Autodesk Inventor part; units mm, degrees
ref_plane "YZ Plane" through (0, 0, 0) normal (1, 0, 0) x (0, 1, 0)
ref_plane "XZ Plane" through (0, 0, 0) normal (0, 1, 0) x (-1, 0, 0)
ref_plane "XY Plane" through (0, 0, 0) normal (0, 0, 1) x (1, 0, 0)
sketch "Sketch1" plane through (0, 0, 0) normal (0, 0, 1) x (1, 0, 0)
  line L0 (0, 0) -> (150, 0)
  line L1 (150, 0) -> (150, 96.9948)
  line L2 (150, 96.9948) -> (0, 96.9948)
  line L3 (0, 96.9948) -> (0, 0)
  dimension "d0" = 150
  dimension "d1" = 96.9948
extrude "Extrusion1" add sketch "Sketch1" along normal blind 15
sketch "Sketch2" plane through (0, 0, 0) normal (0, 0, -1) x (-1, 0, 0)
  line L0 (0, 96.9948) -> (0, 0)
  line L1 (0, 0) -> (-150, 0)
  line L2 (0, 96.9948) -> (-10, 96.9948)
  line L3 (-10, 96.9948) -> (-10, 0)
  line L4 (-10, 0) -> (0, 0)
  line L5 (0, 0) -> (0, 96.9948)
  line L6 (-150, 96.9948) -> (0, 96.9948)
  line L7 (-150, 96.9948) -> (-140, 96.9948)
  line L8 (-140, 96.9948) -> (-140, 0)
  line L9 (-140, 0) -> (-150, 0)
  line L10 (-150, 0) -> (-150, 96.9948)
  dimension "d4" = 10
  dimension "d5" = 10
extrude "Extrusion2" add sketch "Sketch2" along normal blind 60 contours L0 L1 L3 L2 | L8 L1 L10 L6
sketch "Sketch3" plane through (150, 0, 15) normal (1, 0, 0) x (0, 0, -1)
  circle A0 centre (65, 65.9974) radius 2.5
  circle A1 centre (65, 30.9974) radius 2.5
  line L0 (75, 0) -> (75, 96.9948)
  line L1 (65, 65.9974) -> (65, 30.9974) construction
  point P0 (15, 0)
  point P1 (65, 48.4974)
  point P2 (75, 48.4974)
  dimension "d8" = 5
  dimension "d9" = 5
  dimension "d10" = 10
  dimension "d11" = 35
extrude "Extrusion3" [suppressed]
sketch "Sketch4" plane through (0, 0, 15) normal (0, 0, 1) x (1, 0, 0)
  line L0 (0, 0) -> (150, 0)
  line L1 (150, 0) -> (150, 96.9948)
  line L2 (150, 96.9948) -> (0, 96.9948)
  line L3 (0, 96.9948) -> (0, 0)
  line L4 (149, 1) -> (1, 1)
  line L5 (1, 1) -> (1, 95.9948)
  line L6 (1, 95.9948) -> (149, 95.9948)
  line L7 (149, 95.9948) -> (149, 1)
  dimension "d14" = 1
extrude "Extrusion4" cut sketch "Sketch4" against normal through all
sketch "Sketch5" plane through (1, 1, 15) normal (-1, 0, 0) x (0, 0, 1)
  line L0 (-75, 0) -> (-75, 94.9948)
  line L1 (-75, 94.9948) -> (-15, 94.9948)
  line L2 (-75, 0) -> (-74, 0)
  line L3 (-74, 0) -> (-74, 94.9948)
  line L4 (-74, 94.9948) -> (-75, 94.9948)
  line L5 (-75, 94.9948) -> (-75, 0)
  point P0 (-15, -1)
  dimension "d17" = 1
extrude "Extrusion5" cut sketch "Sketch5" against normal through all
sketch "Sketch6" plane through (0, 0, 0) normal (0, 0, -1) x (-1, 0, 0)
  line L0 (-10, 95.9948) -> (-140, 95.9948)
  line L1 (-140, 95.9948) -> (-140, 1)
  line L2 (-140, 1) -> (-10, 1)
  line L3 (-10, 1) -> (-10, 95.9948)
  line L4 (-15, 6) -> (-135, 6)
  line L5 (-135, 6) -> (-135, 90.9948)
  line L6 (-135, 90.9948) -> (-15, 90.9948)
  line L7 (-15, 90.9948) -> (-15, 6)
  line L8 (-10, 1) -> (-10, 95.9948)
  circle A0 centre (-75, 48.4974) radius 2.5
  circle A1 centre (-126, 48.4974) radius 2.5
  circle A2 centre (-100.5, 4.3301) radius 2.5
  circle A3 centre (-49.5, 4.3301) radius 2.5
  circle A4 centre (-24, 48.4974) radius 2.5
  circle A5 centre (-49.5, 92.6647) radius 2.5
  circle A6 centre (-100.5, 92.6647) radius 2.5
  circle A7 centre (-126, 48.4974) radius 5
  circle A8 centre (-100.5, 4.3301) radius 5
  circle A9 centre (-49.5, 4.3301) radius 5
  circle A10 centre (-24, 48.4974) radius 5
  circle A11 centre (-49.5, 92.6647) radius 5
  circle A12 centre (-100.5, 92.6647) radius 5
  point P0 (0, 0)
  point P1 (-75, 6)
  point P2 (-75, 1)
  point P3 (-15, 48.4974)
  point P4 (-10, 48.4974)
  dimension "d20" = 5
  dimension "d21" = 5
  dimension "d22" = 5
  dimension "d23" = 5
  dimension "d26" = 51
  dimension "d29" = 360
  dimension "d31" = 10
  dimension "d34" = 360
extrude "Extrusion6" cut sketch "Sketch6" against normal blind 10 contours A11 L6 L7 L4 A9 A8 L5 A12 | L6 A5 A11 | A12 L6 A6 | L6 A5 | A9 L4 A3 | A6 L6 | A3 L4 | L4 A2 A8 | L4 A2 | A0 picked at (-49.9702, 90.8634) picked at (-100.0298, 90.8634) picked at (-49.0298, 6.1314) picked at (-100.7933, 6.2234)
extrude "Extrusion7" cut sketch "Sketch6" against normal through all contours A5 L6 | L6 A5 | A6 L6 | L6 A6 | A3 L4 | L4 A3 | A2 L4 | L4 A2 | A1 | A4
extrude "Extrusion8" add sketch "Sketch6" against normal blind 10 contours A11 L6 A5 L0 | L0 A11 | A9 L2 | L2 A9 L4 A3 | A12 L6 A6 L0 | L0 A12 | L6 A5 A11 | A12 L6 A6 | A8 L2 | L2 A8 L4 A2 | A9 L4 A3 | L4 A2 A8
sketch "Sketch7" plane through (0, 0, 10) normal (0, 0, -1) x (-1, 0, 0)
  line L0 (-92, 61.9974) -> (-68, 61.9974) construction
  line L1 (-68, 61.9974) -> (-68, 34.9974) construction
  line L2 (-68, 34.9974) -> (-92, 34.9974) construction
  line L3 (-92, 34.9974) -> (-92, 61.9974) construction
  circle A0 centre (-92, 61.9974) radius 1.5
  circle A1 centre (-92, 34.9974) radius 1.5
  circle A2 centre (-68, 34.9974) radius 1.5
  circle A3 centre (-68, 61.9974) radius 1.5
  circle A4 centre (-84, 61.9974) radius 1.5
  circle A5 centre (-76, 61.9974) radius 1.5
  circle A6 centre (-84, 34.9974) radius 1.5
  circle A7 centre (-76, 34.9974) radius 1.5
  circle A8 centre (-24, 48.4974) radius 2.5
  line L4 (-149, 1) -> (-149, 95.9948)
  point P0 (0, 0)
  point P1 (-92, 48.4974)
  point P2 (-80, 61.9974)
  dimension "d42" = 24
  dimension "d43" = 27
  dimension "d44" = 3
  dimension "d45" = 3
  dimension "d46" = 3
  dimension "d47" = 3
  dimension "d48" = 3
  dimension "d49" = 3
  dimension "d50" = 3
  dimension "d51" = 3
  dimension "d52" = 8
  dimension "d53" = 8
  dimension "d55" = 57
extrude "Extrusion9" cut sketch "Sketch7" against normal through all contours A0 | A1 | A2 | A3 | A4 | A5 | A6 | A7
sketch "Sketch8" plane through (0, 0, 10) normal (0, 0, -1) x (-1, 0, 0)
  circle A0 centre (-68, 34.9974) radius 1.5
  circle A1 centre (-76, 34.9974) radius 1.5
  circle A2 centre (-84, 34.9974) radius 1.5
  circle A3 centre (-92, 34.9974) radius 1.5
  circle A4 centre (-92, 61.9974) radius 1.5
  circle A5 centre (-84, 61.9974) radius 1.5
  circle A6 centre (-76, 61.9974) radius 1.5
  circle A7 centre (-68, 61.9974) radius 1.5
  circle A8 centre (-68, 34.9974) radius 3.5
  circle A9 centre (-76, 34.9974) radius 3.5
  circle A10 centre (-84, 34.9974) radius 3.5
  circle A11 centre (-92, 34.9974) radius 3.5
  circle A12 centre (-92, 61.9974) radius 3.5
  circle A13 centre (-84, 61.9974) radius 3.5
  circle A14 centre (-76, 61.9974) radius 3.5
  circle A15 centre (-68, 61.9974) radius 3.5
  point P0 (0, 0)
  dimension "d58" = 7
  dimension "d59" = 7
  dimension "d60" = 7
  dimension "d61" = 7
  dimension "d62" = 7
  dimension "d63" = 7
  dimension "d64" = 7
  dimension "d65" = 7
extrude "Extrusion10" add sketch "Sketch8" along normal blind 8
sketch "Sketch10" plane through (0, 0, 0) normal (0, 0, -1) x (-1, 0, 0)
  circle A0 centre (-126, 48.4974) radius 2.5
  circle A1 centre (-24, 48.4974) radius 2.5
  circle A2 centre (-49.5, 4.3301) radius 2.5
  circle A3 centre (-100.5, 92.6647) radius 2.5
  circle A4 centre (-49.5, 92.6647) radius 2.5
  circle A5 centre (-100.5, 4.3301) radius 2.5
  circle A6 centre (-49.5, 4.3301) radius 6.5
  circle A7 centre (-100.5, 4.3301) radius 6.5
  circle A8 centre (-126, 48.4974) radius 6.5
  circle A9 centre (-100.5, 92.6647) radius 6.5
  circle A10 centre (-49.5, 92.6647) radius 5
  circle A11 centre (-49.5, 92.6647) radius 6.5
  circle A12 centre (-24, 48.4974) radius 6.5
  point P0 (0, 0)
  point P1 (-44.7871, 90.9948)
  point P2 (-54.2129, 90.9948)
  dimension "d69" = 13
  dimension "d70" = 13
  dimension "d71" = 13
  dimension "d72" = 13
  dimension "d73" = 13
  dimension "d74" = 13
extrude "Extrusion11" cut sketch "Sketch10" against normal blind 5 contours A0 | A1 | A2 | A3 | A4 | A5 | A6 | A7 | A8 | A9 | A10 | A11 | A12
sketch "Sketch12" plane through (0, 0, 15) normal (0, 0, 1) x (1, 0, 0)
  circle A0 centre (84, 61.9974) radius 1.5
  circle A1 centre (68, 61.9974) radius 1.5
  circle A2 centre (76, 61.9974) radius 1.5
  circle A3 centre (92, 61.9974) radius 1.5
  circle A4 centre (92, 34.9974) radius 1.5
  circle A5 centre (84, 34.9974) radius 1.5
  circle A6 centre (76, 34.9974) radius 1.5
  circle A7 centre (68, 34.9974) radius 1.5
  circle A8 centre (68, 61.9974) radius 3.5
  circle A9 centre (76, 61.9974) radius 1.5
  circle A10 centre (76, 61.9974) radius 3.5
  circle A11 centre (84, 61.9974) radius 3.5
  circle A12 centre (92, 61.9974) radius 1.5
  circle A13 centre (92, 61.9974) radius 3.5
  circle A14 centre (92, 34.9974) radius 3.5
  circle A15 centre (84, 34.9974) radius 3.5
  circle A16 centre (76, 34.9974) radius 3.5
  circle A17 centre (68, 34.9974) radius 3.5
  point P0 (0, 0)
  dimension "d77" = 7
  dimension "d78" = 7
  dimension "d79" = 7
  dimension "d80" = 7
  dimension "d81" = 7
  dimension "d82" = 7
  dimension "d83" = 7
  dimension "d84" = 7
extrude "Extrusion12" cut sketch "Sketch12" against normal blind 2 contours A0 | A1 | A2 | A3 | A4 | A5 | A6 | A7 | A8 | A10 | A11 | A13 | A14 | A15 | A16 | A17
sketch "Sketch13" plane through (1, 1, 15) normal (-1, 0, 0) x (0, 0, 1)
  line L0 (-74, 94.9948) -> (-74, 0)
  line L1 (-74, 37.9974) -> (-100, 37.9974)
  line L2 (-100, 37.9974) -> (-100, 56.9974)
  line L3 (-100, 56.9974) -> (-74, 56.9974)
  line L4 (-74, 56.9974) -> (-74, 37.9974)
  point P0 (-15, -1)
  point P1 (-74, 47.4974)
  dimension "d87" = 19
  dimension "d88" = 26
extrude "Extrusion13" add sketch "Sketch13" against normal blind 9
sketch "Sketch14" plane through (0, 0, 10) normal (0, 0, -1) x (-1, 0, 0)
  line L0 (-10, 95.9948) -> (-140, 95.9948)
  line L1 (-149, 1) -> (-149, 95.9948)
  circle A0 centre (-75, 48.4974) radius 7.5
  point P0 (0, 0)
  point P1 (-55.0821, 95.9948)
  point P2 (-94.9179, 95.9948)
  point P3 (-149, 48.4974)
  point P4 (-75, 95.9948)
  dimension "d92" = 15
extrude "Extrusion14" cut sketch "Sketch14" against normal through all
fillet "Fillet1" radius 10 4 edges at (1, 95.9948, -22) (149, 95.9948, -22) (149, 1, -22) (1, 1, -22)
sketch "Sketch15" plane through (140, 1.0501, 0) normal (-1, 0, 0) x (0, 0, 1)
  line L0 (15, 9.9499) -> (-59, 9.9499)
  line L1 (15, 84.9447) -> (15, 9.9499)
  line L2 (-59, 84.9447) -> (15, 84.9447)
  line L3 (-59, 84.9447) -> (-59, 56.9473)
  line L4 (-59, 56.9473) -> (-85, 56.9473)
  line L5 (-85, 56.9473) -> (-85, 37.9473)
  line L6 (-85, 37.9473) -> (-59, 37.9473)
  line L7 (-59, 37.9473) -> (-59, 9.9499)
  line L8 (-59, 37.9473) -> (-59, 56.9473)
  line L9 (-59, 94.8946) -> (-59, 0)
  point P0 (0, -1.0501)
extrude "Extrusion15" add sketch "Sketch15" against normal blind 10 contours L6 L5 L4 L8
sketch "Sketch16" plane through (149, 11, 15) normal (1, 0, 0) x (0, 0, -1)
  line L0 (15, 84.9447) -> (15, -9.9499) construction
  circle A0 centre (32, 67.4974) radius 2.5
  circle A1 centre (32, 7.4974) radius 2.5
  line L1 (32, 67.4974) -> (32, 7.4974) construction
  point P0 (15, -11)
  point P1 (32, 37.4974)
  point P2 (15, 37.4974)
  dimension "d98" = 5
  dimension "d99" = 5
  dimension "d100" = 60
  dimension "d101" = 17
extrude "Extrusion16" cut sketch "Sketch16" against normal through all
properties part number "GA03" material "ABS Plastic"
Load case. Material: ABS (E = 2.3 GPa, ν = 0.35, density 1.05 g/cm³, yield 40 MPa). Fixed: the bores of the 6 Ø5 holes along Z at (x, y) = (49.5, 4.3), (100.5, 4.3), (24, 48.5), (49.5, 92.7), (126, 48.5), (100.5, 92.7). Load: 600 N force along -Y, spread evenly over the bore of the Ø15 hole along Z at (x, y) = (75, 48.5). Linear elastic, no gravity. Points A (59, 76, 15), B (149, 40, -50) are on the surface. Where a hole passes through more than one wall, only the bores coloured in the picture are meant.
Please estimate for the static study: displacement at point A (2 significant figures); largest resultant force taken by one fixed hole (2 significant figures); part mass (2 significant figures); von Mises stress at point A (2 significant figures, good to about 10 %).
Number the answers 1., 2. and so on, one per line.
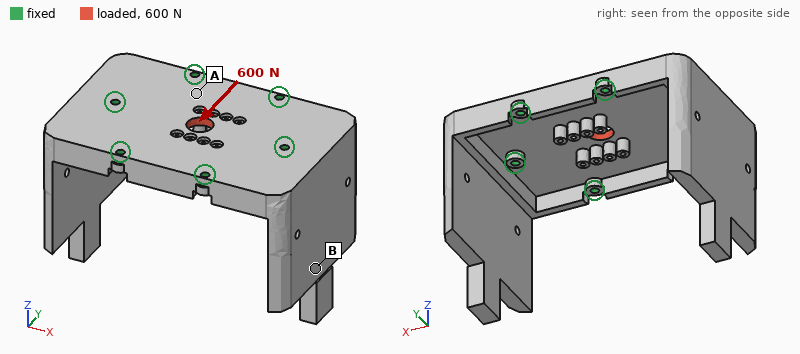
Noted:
1. 12 µm
2. 140 N
3. 220 g
4. 1.2 MPa
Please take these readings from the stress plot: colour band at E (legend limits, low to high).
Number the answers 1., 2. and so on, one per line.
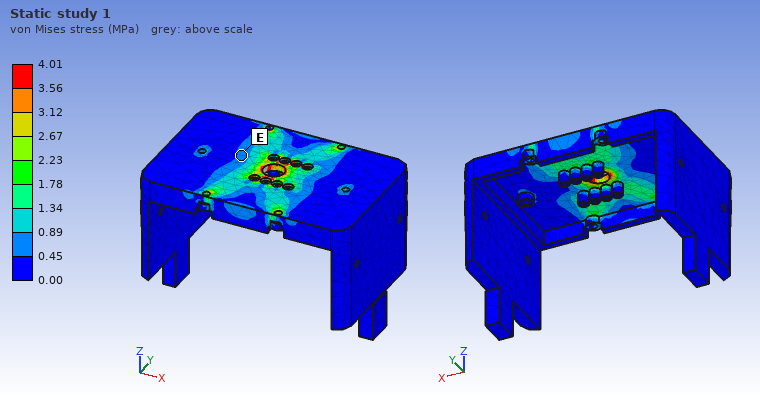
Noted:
1. 0.45 to 0.89 MPa
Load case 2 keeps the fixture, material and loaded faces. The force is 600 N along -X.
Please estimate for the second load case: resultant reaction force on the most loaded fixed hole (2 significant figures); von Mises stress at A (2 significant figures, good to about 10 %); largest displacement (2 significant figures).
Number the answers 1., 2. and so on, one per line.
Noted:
1. 150 N
2. 0.58 MPa
3. 34 µm
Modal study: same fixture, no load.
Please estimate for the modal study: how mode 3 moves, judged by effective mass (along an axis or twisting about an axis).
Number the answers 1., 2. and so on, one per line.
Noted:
1. along Y
